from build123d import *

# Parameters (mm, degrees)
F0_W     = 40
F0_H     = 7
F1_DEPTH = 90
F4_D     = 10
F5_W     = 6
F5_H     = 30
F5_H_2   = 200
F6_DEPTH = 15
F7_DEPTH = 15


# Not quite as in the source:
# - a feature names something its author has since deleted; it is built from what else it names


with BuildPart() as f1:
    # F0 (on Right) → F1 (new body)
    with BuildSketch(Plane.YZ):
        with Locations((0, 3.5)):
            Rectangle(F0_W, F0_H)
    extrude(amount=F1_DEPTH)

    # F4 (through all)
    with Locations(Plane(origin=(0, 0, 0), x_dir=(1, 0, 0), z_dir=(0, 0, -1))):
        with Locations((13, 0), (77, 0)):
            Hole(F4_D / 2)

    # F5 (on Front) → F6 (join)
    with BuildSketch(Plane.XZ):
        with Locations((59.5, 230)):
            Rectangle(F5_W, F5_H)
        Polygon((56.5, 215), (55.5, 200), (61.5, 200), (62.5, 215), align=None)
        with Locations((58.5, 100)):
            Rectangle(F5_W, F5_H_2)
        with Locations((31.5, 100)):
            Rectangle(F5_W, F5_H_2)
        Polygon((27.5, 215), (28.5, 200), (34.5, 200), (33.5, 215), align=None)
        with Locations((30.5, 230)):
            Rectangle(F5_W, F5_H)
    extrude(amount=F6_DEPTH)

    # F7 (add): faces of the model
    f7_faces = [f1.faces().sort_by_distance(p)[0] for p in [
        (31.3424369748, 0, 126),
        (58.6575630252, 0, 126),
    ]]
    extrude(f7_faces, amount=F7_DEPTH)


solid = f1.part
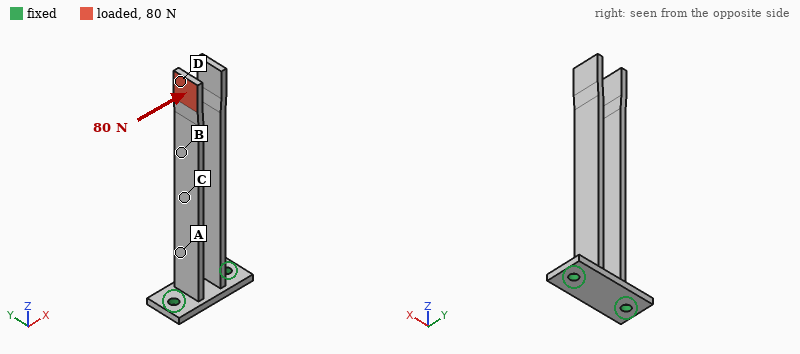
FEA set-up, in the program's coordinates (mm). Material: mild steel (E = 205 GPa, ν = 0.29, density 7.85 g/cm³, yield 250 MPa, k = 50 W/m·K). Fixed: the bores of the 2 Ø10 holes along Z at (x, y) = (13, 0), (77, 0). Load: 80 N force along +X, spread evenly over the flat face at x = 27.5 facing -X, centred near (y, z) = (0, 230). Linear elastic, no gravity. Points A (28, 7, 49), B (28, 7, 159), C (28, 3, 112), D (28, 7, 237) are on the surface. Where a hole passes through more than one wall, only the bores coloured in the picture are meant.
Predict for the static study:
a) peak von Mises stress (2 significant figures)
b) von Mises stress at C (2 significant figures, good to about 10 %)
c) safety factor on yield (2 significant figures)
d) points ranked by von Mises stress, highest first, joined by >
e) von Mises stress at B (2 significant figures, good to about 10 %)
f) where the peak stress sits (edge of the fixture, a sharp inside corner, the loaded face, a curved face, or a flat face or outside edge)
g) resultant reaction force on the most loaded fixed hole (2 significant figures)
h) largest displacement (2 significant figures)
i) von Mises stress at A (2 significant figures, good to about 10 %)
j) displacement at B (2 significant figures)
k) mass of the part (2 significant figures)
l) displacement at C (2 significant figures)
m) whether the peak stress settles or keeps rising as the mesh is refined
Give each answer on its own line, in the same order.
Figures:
99 MPa
53 MPa
2.5
A > C > B > D
31 MPa
a flat face or outside edge
360 N
3.1 mm
80 MPa
1.5 mm
860 g
0.80 mm
settles
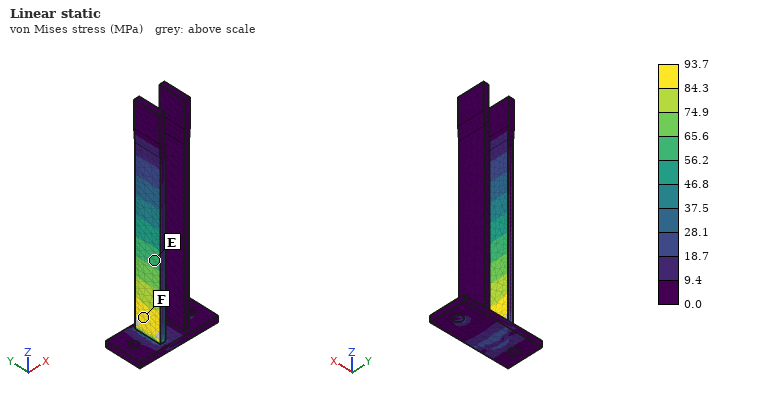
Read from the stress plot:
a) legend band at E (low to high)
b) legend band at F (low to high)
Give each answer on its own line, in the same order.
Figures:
56.2 to 65.6 MPa
84.3 to 93.7 MPa
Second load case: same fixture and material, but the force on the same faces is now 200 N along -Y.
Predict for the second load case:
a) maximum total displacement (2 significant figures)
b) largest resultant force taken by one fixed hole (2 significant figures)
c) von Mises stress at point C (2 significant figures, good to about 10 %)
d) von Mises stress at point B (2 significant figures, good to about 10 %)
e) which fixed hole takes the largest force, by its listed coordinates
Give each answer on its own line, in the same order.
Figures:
0.56 mm
160 N
8.7 MPa
9.8 MPa
(13, 0)
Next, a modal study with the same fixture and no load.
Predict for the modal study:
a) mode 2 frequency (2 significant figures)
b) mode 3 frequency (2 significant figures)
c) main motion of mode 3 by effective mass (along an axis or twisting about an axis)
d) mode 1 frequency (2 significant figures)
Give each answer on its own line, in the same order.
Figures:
86 Hz
260 Hz
along Y
84 Hz
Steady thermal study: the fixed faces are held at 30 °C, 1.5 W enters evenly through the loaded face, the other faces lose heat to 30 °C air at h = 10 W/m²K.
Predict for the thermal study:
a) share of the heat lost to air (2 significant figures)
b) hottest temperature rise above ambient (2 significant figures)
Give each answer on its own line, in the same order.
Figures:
78 %
17 K
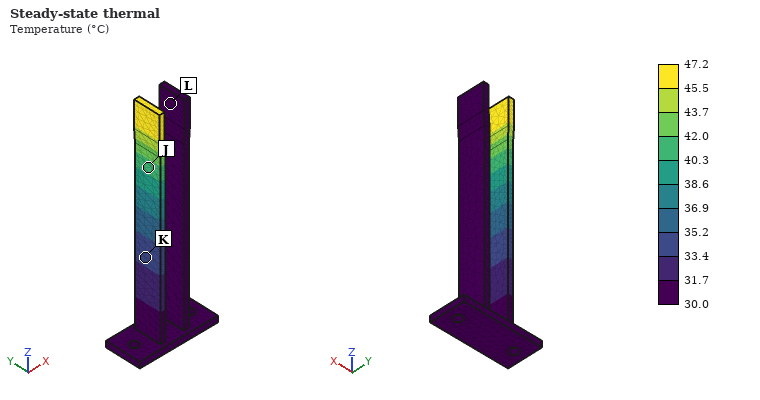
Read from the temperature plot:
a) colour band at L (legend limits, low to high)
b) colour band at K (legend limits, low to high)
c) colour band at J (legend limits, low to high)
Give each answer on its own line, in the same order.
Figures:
30.0 to 31.7 °C
33.4 to 35.2 °C
40.3 to 42.0 °C
